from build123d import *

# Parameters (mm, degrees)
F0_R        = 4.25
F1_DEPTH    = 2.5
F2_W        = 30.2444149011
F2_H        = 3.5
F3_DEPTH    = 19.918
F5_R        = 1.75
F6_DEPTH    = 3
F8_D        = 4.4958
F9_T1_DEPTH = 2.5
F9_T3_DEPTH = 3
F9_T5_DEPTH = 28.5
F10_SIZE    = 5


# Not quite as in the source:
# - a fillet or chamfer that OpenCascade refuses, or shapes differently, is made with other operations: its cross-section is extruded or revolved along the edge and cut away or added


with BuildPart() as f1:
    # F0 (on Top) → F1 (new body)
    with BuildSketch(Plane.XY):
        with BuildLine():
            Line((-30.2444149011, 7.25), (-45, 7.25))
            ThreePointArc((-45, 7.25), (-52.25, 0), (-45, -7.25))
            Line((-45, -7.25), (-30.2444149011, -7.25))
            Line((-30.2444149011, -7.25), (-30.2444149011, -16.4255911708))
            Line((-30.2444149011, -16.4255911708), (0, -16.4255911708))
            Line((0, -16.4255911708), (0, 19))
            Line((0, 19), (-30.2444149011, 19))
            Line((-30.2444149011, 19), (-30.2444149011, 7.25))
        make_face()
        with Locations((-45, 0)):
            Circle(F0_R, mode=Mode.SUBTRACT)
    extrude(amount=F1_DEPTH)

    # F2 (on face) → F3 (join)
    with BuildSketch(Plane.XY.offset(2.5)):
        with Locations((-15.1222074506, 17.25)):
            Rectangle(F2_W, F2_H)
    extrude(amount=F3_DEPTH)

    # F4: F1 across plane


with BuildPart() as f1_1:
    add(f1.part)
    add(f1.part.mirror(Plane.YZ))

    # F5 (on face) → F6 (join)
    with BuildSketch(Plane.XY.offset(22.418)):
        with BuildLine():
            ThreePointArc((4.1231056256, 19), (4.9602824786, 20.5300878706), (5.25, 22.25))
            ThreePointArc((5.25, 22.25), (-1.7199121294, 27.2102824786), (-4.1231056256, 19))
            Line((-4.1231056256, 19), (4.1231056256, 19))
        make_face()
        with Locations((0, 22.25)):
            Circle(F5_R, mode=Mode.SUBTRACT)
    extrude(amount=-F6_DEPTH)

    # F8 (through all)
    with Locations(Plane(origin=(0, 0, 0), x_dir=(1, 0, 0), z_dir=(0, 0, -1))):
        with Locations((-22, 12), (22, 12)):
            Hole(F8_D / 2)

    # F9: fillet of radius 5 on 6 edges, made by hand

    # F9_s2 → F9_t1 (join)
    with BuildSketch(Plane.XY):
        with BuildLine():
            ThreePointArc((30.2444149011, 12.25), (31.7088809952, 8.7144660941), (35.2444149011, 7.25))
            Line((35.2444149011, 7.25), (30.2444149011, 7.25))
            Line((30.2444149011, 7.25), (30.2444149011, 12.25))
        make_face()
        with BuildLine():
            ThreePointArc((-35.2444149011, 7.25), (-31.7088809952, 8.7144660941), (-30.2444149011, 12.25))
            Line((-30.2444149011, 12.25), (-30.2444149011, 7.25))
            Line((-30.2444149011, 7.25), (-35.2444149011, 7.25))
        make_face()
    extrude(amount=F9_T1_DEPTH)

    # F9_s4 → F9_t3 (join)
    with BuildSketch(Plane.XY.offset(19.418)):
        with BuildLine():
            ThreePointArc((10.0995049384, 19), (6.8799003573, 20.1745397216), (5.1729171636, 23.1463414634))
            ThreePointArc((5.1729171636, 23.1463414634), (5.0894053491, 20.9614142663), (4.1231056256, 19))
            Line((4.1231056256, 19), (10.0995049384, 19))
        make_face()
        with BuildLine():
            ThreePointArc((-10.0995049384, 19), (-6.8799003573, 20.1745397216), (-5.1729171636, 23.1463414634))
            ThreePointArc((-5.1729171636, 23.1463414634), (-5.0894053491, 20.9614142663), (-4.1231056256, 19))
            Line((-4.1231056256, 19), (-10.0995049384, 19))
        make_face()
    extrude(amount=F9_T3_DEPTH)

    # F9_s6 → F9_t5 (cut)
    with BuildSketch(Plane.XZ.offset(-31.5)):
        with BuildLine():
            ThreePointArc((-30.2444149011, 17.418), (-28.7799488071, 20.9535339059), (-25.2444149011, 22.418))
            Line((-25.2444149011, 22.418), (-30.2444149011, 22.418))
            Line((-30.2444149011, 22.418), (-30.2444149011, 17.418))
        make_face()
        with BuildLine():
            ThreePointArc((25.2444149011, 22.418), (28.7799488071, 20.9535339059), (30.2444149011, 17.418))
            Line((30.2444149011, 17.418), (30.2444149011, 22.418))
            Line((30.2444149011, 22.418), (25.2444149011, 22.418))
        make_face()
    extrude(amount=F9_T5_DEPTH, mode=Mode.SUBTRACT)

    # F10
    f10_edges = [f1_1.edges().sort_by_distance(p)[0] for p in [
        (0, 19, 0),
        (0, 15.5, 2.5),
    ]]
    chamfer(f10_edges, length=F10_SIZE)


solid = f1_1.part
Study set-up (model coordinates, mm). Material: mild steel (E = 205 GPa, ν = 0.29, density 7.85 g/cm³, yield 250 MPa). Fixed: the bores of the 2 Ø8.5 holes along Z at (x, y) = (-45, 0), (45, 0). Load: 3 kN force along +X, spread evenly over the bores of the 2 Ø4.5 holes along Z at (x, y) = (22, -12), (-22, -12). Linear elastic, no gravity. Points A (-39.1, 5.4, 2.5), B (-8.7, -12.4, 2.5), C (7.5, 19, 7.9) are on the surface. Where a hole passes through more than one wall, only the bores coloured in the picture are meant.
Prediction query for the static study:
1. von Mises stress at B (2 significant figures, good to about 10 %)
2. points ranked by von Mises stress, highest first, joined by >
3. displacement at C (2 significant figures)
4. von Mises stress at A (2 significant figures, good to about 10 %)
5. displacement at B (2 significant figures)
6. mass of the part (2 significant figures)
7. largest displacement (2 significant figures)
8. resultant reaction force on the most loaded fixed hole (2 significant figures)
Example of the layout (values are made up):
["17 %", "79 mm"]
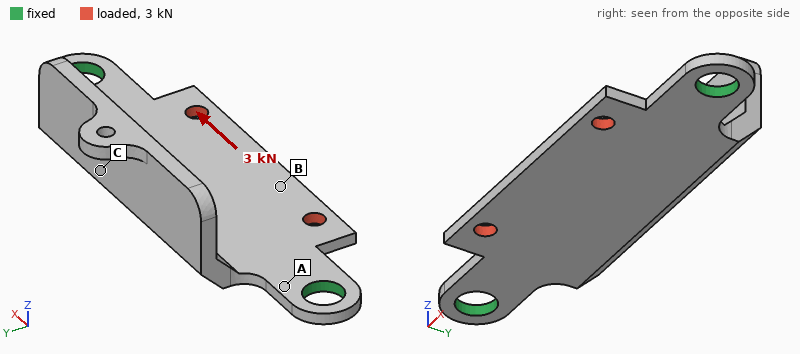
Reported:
["18 MPa", "A > B > C", "2.0 µm", "35 MPa", "6.6 µm", "86 g", "11 µm", "1.6 kN"]
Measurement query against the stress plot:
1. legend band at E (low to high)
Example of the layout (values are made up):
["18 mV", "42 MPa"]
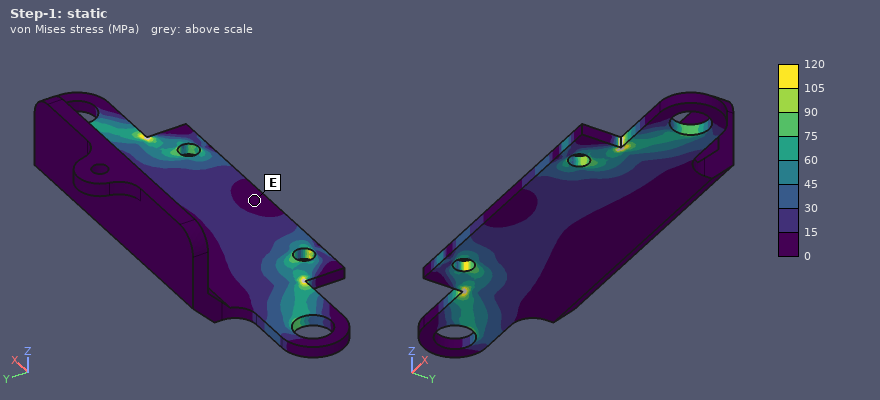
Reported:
["0 to 15 MPa"]
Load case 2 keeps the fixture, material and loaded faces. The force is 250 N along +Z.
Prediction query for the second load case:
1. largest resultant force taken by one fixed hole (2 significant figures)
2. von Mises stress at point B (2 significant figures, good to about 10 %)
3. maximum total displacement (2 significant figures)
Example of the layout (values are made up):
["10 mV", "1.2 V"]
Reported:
["130 N", "17 MPa", "0.12 mm"]
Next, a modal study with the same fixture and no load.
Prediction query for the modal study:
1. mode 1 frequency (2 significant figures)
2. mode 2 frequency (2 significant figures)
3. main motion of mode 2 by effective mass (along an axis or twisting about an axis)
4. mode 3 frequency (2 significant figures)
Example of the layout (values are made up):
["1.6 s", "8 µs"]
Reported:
["990 Hz", "2000 Hz", "along Z", "3100 Hz"]
